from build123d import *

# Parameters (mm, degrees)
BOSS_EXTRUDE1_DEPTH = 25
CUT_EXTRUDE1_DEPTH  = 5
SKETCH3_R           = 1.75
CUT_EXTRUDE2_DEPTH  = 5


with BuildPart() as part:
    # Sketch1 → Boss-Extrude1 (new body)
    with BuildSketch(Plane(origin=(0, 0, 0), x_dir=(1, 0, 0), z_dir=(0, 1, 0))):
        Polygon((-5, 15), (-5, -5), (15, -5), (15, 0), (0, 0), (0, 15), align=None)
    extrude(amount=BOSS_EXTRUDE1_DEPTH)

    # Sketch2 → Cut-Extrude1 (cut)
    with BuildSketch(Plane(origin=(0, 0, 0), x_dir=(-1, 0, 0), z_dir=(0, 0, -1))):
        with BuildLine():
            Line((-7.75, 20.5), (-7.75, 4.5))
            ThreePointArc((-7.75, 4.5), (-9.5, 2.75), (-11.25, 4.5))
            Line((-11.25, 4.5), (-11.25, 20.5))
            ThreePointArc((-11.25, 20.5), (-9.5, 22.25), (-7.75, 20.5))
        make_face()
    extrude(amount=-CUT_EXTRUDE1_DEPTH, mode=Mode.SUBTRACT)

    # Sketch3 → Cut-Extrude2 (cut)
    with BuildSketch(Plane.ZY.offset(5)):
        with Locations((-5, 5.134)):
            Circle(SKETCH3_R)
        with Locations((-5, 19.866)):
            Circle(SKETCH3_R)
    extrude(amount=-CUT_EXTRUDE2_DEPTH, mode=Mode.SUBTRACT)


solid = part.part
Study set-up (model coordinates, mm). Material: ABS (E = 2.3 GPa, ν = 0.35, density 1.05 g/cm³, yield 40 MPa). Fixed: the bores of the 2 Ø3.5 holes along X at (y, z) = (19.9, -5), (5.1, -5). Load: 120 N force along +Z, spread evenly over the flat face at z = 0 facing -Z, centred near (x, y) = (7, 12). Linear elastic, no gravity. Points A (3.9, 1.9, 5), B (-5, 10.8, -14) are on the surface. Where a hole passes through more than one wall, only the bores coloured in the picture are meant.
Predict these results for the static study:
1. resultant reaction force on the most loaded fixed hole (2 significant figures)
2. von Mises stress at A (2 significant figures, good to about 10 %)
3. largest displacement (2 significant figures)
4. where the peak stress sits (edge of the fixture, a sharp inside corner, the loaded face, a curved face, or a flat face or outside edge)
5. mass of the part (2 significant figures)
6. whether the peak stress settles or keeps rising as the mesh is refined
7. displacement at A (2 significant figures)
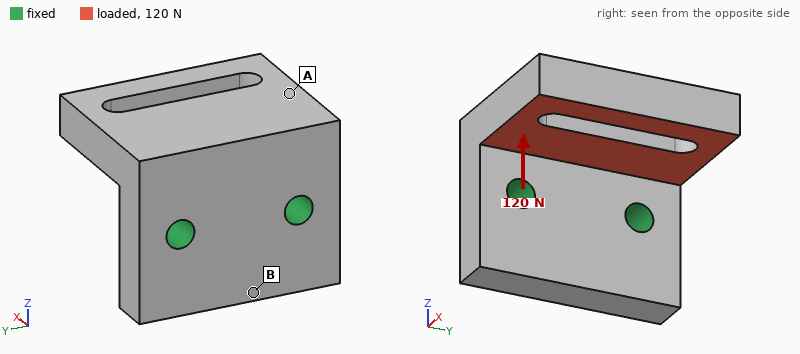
61 N
7.3 MPa
0.45 mm
edge of the fixture
4.1 g
keeps rising
0.14 mm
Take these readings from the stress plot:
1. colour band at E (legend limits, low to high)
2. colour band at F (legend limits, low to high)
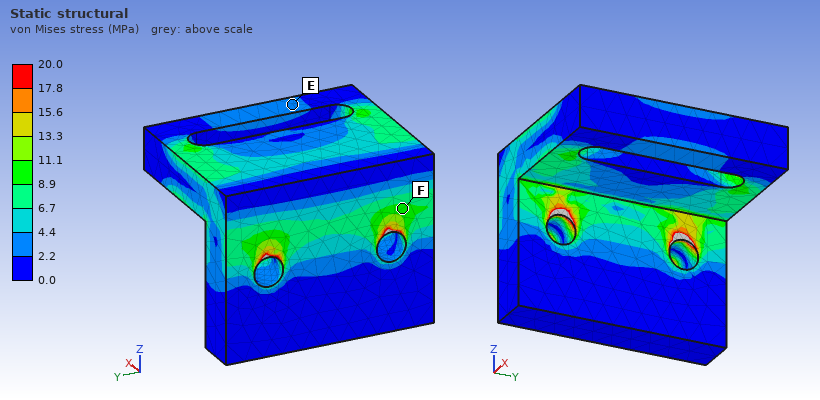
2.2 to 4.4 MPa
8.9 to 11.1 MPa
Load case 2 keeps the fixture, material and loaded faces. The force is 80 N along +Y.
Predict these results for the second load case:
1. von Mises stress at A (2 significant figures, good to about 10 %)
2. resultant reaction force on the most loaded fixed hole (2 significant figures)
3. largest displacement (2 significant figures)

1.9 MPa
61 N
0.11 mm
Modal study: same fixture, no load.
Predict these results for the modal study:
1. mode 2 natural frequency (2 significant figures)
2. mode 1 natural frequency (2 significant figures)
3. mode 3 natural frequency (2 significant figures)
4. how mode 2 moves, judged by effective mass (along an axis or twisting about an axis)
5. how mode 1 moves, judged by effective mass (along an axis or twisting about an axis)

4300 Hz
2500 Hz
5600 Hz
along Y
along Z
